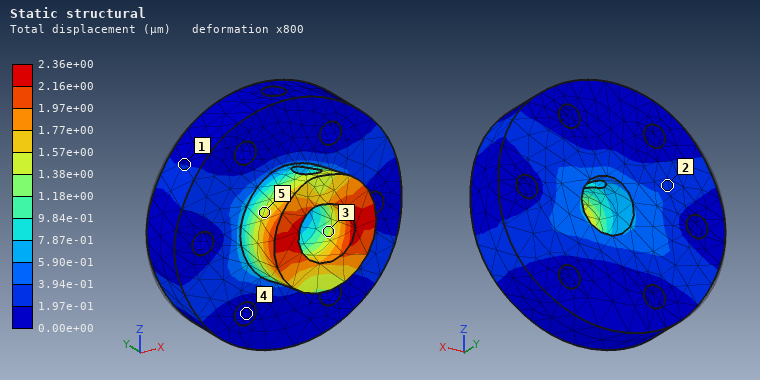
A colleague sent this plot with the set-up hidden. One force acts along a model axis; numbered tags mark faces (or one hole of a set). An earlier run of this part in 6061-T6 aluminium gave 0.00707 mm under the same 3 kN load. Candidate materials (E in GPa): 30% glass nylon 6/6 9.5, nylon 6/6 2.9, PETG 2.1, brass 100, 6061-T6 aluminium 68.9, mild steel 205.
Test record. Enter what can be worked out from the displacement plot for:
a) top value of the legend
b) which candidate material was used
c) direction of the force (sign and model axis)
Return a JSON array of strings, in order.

["2.36e+00 µm", "mild steel", "+X"]
